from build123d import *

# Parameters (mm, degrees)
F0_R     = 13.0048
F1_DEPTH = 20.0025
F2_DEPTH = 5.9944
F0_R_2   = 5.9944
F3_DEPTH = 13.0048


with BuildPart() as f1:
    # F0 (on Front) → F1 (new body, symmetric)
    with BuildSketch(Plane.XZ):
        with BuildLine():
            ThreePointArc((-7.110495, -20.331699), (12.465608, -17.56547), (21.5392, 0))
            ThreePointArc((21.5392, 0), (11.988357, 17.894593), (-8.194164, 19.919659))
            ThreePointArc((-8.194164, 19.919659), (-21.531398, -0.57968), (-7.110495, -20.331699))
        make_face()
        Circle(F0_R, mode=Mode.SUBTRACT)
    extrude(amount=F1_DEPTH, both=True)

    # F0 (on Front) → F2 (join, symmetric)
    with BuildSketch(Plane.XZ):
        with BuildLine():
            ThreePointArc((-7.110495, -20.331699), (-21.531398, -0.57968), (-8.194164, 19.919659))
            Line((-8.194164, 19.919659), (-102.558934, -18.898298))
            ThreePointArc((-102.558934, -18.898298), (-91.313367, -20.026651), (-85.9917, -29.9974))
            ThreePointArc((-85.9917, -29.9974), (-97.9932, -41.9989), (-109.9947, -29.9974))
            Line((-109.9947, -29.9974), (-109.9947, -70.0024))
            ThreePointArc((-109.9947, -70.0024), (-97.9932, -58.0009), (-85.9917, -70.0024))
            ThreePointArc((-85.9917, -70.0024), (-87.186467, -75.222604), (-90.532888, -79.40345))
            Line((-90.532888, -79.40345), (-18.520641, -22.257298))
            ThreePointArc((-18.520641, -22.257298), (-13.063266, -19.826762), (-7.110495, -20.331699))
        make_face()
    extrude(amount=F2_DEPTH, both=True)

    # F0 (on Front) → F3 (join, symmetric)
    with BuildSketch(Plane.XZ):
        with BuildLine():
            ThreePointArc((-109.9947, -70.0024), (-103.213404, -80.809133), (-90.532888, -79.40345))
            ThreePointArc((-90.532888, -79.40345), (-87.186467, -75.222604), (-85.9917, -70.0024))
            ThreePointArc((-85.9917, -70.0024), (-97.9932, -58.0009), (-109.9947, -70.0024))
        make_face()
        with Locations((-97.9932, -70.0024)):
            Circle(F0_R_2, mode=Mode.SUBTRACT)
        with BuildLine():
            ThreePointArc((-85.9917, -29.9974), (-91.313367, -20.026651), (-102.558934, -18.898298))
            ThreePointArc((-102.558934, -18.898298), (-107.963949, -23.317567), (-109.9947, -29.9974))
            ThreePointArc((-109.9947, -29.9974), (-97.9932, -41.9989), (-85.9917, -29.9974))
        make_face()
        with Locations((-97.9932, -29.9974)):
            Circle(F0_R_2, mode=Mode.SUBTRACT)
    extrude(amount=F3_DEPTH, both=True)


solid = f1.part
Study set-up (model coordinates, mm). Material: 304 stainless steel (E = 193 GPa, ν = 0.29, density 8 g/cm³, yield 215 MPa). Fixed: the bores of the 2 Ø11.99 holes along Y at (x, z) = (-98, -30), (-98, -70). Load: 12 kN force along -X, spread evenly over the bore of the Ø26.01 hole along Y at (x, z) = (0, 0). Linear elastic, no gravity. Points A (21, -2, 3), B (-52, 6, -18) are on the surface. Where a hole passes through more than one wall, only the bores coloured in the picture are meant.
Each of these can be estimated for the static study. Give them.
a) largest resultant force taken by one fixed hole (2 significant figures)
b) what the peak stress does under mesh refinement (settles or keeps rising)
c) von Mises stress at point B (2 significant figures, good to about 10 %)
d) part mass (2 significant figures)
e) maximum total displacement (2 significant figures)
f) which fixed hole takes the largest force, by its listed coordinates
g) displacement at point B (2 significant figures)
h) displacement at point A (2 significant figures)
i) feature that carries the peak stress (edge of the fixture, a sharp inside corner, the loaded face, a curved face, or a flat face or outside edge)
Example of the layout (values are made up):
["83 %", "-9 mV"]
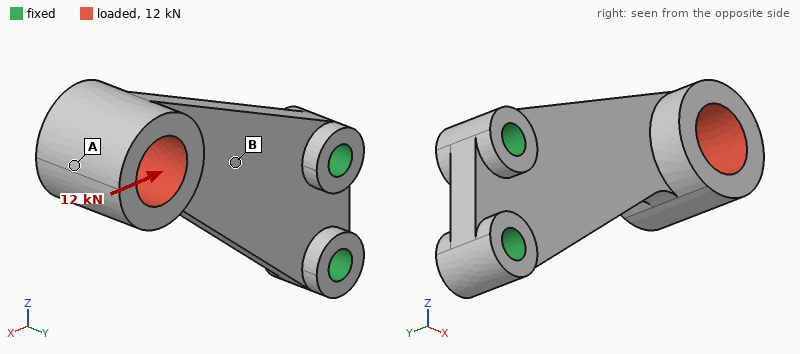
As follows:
["19 kN", "keeps rising", "37 MPa", "820 g", "0.12 mm", "(-98, -30)", "0.024 mm", "0.12 mm", "edge of the fixture"]
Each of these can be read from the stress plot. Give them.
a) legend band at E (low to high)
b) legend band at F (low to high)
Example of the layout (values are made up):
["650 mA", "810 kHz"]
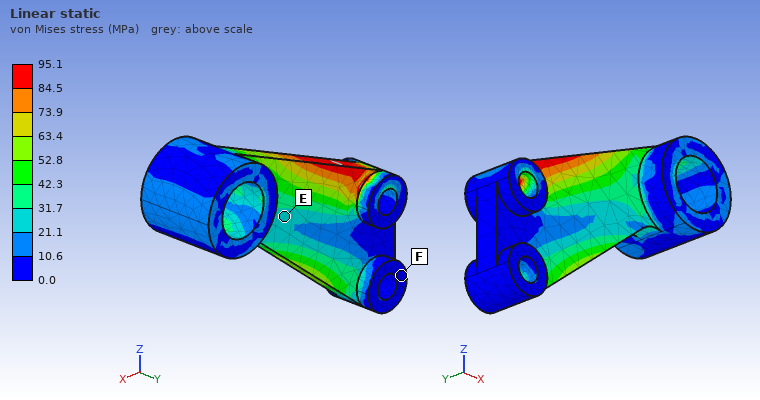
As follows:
["21.1 to 31.7 MPa", "0.0 to 10.6 MPa"]
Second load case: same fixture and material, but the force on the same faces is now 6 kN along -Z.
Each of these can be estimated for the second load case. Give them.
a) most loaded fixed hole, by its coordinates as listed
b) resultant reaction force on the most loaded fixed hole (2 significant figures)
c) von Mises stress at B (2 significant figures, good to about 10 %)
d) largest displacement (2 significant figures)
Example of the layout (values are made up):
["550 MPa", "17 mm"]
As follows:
["(-98, -70)", "14 kN", "17 MPa", "0.16 mm"]
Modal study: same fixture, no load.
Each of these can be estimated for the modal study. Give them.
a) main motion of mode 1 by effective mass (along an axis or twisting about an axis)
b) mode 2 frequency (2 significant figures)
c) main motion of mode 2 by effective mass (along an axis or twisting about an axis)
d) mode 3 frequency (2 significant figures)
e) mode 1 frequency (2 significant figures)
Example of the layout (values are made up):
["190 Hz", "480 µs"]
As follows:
["along Y", "1900 Hz", "along Z", "2300 Hz", "550 Hz"]
